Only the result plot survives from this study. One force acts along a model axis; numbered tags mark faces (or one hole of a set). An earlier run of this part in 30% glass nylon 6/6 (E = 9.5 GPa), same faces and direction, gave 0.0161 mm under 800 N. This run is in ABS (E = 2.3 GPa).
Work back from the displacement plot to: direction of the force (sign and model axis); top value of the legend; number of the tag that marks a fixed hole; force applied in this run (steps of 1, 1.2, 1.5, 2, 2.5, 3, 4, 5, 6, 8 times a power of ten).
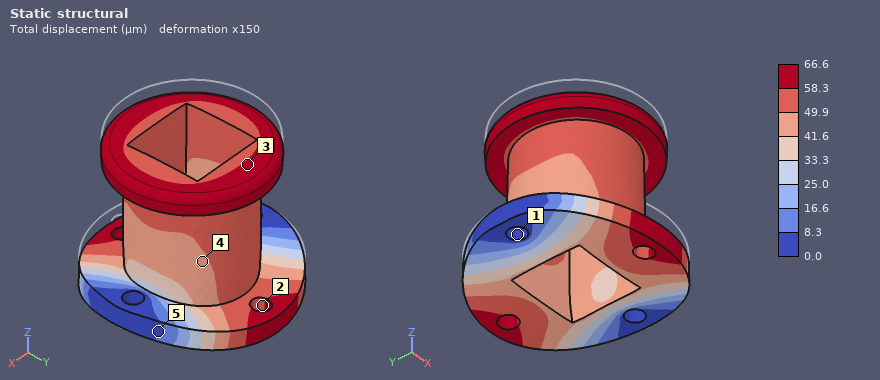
-Z
66.6 µm
1
800 N
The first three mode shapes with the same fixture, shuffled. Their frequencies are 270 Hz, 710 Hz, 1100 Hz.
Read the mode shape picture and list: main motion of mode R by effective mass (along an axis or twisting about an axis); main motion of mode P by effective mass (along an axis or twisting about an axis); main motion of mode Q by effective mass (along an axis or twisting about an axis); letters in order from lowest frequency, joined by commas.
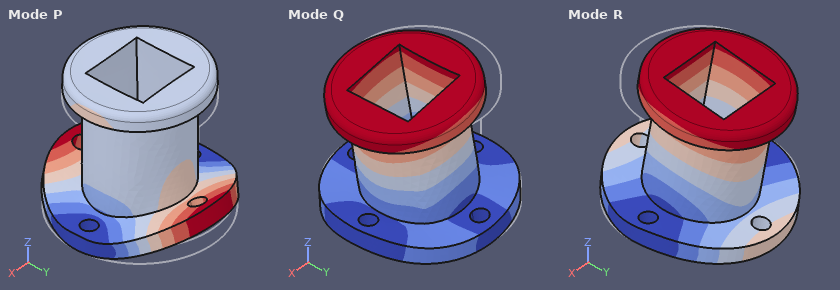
along Y
along Z
along X
R, Q, P
